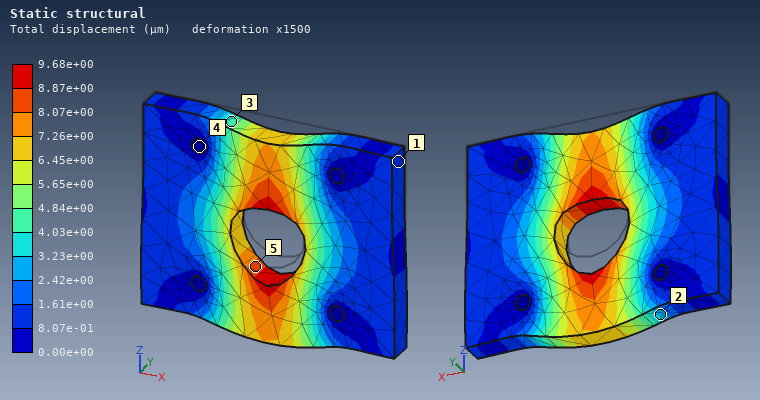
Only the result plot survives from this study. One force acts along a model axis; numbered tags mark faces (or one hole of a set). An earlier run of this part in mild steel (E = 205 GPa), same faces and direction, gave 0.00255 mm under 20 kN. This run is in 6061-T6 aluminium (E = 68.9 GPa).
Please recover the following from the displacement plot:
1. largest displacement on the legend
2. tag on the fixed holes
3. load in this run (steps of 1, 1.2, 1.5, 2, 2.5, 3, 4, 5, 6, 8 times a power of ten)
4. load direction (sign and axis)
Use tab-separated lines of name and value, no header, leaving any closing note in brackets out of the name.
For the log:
largest displacement on the legend	9.68e+00 µm
tag on the fixed holes	4
load in this run	25 kN
load direction	-Z
